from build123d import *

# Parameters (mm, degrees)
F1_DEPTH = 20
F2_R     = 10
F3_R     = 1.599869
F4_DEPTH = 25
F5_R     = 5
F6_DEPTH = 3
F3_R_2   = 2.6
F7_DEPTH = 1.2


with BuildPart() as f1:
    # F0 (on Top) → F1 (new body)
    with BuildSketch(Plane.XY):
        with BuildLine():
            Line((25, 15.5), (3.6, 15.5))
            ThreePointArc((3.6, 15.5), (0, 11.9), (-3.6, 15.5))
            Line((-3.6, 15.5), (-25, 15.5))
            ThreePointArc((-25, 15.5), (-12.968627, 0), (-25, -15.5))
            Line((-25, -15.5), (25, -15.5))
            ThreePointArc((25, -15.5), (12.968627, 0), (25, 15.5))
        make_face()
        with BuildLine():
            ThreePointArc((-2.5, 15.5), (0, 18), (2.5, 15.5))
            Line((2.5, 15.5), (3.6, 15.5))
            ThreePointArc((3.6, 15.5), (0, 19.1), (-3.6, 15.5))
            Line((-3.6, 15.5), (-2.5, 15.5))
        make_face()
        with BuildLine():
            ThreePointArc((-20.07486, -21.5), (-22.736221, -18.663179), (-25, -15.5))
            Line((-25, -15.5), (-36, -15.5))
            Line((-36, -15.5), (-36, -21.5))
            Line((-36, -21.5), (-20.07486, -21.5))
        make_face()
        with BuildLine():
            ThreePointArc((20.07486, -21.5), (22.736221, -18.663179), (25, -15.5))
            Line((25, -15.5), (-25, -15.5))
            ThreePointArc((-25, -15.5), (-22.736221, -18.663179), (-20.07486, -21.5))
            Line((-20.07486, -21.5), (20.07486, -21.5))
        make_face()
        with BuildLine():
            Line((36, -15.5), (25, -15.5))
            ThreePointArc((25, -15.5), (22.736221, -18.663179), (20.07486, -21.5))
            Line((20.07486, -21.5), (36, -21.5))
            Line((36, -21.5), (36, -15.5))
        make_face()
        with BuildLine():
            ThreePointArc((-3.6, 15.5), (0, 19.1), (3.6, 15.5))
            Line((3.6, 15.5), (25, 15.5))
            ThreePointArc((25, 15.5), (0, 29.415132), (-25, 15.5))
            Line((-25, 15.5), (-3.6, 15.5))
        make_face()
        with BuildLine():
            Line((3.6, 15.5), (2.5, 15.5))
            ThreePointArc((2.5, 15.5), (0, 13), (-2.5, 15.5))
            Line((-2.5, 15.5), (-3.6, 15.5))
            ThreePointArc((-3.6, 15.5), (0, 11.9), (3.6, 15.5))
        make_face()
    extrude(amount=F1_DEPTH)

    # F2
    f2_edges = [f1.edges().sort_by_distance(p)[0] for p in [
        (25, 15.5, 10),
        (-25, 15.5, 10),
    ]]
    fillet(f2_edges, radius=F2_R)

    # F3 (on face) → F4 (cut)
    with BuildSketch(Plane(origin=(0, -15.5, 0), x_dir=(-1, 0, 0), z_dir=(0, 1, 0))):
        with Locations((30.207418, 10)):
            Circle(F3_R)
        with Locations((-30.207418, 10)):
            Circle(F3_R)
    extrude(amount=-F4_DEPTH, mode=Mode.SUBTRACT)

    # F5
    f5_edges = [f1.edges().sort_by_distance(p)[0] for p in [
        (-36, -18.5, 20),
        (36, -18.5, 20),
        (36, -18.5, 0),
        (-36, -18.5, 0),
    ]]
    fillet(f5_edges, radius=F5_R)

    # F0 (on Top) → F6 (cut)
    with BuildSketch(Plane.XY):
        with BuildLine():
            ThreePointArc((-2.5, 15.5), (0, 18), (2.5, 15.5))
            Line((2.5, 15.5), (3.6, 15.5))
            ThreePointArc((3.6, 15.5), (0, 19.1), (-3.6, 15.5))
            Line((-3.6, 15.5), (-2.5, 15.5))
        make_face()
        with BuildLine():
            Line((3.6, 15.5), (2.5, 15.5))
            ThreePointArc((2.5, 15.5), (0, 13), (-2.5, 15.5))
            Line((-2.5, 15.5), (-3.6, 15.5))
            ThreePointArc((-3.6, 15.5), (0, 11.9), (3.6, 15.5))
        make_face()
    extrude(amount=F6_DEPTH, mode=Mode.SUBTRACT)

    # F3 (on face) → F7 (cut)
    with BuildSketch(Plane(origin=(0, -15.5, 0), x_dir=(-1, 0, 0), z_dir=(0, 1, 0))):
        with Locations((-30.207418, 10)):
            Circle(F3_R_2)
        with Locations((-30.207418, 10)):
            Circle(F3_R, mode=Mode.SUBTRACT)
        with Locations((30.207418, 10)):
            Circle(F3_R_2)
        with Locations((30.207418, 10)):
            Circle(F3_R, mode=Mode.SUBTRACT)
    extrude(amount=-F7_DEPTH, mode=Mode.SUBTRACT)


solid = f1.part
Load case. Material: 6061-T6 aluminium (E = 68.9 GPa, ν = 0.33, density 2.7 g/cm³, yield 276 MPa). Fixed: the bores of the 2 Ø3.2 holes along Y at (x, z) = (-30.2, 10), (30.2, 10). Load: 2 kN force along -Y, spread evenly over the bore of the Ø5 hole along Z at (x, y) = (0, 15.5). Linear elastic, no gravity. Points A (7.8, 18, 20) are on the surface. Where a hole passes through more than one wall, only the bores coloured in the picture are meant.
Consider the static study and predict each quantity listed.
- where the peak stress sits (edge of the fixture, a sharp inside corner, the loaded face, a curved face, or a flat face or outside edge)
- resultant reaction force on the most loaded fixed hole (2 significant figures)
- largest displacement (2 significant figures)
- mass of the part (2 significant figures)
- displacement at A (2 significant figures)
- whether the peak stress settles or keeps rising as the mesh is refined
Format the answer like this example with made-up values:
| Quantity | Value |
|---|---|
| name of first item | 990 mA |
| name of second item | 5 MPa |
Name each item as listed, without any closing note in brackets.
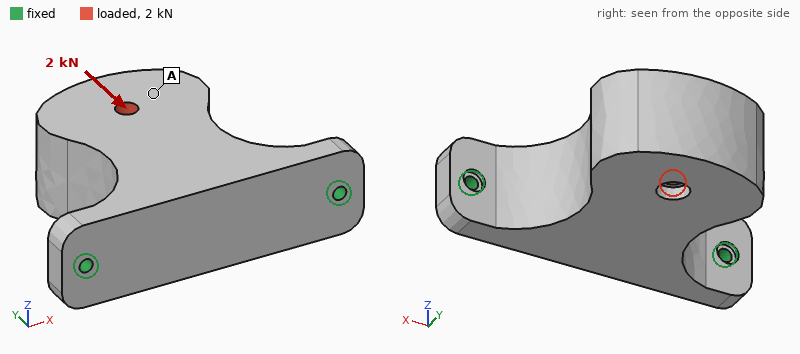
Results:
| Quantity | Value |
|---|---|
| where the peak stress sits | edge of the fixture |
| resultant reaction force on the most loaded fixed hole | 1.3 kN |
| largest displacement | 44 µm |
| mass of the part | 98 g |
| displacement at A | 37 µm |
| whether the peak stress settles or keeps rising as the mesh is refined | keeps rising |
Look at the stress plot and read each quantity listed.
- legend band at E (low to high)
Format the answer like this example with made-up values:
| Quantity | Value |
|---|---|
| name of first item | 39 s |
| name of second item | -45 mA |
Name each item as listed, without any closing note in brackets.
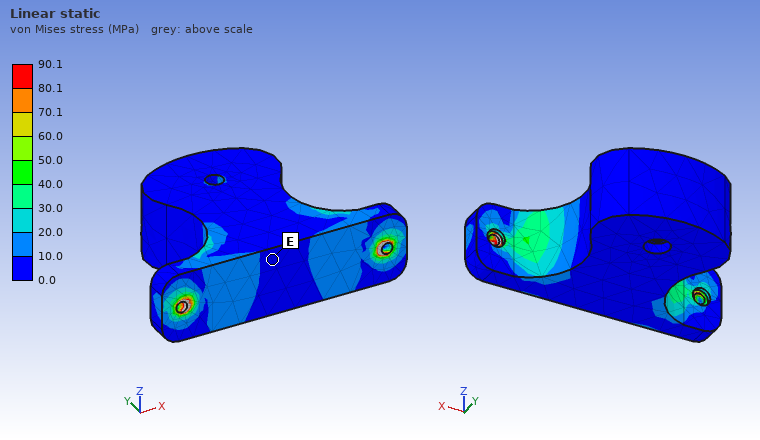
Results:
| Quantity | Value |
|---|---|
| legend band at E | 0.0 to 10.0 MPa |
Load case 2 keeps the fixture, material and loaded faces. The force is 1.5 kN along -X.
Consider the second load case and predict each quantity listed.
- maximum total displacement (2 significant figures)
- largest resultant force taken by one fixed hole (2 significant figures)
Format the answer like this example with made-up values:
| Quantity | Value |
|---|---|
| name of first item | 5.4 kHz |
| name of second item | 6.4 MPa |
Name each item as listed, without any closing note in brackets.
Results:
| Quantity | Value |
|---|---|
| maximum total displacement | 40 µm |
| largest resultant force taken by one fixed hole | 1.2 kN |
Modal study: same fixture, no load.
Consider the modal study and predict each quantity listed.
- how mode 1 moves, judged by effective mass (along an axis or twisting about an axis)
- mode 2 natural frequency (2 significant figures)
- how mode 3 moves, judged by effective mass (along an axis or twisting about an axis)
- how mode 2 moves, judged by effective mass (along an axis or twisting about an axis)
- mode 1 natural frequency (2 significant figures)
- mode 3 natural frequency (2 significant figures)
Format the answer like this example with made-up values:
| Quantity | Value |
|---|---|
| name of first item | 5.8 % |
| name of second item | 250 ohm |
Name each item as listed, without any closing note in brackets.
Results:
| Quantity | Value |
|---|---|
| how mode 1 moves, judged by effective mass | along Z |
| mode 2 natural frequency | 4900 Hz |
| how mode 3 moves, judged by effective mass | along Y |
| how mode 2 moves, judged by effective mass | along X |
| mode 1 natural frequency | 1300 Hz |
| mode 3 natural frequency | 5600 Hz |
